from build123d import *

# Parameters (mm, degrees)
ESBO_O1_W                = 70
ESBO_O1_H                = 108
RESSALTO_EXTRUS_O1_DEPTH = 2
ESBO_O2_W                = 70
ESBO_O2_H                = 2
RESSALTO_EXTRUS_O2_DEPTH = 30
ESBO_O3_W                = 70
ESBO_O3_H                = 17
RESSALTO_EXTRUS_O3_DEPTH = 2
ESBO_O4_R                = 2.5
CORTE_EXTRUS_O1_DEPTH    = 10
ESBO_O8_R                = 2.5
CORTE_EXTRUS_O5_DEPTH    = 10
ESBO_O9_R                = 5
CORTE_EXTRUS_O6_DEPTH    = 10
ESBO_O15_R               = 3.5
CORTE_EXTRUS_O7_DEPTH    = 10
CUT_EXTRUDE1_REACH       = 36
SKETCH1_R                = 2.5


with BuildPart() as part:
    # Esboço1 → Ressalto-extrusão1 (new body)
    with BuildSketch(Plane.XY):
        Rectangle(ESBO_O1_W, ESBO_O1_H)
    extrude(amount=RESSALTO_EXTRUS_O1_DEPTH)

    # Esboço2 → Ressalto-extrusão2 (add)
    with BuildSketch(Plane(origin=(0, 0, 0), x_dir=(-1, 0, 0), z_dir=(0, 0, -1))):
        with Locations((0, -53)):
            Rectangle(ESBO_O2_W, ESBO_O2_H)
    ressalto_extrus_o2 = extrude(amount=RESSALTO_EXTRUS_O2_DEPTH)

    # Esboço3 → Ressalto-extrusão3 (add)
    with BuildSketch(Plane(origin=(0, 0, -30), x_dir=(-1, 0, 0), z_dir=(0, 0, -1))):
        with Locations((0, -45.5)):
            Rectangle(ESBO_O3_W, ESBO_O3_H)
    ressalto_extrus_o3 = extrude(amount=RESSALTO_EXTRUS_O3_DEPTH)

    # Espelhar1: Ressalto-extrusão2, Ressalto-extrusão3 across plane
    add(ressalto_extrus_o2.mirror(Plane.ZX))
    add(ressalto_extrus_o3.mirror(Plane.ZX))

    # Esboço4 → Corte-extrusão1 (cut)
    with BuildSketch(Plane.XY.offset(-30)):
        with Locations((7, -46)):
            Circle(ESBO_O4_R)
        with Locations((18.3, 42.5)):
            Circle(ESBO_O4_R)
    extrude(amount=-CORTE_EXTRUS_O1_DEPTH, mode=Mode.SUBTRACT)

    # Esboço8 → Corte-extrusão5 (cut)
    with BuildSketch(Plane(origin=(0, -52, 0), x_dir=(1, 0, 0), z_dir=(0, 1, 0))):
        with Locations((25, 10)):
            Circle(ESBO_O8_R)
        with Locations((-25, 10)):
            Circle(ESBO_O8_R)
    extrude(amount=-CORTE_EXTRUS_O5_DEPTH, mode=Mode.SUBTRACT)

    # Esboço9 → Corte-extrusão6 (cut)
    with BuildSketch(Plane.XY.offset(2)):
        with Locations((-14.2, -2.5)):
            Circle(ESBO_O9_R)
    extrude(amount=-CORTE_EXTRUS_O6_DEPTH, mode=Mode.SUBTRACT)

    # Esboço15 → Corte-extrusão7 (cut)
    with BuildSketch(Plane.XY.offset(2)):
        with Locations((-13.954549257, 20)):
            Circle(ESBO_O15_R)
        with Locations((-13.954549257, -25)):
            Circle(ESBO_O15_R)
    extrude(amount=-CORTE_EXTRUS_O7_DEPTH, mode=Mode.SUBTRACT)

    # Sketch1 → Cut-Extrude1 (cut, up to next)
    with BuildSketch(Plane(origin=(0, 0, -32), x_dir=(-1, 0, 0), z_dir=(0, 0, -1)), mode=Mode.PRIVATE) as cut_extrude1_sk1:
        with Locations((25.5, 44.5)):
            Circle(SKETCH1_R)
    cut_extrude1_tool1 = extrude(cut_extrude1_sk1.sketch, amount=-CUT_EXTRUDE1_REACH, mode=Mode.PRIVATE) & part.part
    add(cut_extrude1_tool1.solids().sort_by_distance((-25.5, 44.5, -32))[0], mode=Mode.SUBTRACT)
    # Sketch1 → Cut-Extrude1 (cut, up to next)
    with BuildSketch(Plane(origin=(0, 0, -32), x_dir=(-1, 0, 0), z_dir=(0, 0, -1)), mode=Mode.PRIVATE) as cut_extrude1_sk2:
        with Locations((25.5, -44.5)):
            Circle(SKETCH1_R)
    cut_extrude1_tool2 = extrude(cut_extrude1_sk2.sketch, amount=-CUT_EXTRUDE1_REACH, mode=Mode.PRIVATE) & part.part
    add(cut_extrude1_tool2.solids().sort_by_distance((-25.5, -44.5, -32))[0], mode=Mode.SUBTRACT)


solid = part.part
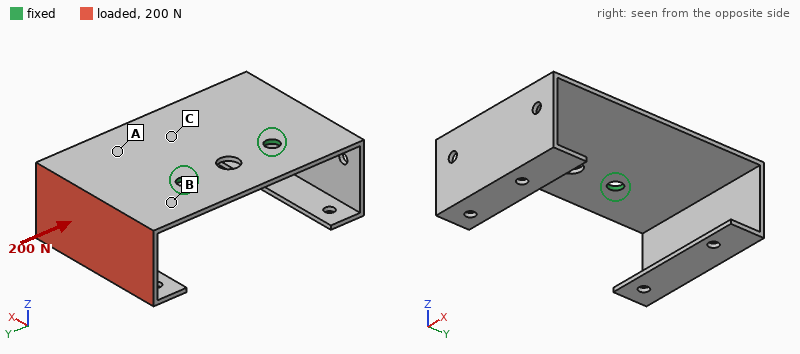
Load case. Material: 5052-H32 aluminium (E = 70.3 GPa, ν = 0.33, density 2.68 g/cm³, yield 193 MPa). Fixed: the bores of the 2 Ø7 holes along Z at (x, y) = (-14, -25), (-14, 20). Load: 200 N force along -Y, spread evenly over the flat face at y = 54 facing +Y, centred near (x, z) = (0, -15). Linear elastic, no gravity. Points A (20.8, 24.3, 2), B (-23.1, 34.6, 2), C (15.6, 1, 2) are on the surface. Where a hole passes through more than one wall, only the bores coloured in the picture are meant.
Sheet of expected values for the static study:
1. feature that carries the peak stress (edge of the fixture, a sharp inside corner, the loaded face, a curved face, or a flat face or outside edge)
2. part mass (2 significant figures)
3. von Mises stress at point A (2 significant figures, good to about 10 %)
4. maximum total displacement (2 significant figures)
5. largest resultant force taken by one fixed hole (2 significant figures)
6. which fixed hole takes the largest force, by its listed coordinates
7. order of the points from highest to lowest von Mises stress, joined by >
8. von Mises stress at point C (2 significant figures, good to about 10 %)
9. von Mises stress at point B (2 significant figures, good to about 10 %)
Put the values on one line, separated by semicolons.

a flat face or outside edge; 74 g; 44 MPa; 1.5 mm; 160 N; (-14, 20); B > A > C; 13 MPa; 71 MPa
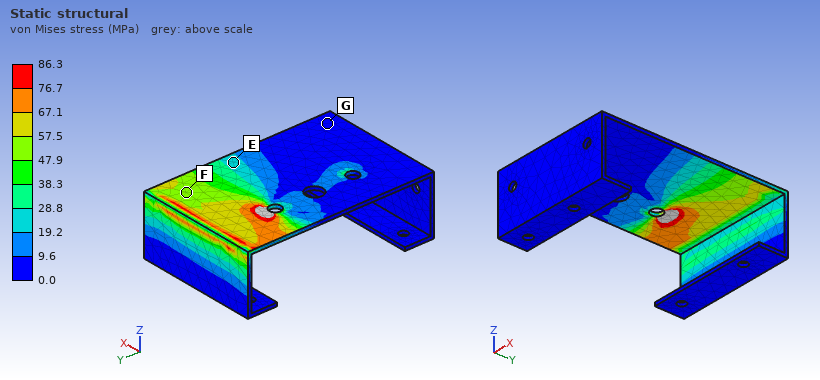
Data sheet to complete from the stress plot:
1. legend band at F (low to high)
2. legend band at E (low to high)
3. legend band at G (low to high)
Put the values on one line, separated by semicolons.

47.9 to 57.5 MPa; 19.2 to 28.8 MPa; 0.0 to 9.6 MPa
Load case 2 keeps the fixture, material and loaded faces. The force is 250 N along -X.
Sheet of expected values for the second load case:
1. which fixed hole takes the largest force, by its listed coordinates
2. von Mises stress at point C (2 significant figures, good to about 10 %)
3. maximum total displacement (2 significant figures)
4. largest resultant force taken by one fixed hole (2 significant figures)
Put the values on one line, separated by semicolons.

(-14, 20); 31 MPa; 1.4 mm; 410 N
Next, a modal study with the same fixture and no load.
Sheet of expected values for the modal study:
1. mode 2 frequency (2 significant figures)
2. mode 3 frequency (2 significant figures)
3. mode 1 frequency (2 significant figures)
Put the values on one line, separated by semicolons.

390 Hz; 440 Hz; 350 Hz
